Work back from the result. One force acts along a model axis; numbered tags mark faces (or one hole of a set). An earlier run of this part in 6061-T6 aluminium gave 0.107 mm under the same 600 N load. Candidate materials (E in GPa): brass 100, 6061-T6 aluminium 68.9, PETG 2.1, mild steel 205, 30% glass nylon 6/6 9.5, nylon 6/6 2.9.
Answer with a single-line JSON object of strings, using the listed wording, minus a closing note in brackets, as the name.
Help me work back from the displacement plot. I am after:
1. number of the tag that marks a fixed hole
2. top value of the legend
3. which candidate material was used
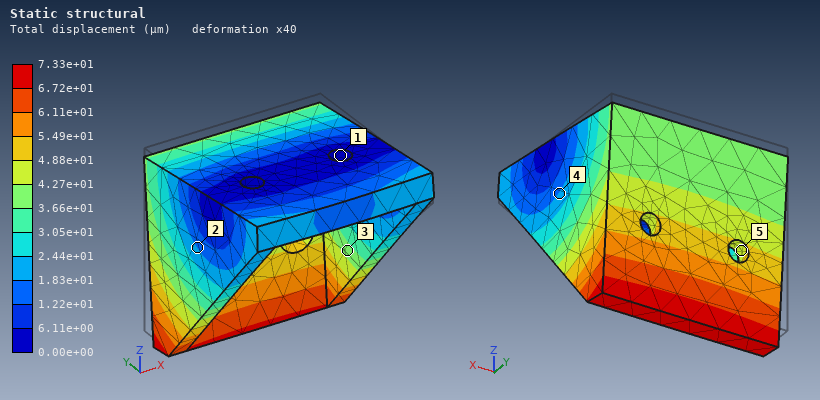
{"number of the tag that marks a fixed hole": "1", "top value of the legend": "7.33e+01 µm", "which candidate material was used": "brass"}
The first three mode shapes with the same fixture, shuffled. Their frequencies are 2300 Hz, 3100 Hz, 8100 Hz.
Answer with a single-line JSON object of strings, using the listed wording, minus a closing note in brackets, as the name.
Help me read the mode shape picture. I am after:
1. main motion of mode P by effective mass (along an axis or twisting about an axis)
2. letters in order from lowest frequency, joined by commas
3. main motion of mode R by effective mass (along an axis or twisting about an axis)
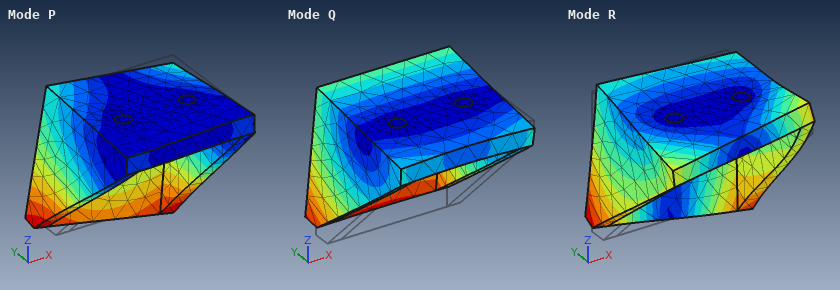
{"main motion of mode P by effective mass": "along X", "letters in order from lowest frequency, joined by commas": "Q, P, R", "main motion of mode R by effective mass": "along X"}
